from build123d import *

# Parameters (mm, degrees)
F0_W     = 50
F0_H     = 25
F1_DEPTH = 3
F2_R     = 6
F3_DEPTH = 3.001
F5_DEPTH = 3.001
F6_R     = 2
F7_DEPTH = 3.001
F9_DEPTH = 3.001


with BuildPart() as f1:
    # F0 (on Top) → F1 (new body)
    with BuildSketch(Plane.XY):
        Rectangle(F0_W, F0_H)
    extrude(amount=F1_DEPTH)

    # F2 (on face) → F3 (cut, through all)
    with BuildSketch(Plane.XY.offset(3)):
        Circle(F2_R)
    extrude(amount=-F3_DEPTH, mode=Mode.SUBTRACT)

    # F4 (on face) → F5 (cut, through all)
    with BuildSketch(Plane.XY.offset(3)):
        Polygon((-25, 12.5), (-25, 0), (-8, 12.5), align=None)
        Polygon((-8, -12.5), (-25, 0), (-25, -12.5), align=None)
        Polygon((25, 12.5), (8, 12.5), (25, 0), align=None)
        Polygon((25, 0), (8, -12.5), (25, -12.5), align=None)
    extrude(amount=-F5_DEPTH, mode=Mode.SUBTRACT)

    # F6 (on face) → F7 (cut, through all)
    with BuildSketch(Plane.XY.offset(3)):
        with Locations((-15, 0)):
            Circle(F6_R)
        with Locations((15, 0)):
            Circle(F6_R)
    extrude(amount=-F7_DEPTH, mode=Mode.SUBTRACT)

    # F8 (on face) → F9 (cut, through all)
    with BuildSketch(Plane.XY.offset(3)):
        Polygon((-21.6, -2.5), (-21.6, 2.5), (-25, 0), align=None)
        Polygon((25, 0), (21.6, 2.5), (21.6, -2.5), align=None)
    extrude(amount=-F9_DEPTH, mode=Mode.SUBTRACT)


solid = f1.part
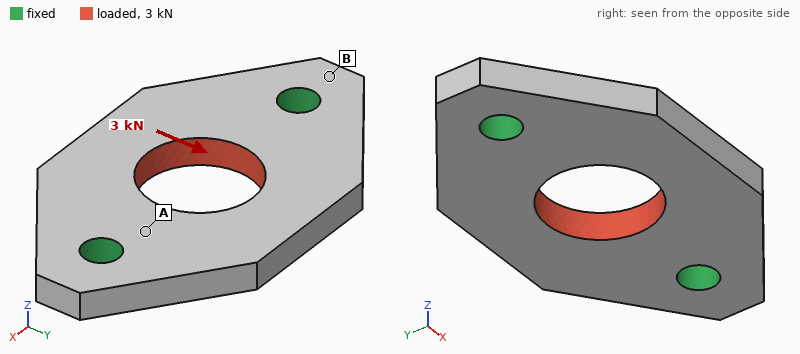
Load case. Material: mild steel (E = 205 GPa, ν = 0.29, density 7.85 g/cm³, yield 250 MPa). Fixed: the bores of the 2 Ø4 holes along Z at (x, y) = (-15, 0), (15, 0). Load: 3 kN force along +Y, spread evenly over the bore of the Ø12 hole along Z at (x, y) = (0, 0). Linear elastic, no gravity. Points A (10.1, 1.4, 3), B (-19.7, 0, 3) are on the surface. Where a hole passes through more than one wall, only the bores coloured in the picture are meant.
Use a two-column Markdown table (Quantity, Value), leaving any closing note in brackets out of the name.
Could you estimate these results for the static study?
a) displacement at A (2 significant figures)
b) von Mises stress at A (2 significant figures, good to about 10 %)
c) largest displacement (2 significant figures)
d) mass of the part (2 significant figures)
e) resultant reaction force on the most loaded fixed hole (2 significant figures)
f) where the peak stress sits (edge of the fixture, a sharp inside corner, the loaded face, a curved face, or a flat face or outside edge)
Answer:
| Quantity | Value |
|---|---|
| displacement at A | 2.2 µm |
| von Mises stress at A | 55 MPa |
| largest displacement | 5.6 µm |
| mass of the part | 16 g |
| resultant reaction force on the most loaded fixed hole | 1.5 kN |
| where the peak stress sits | edge of the fixture |
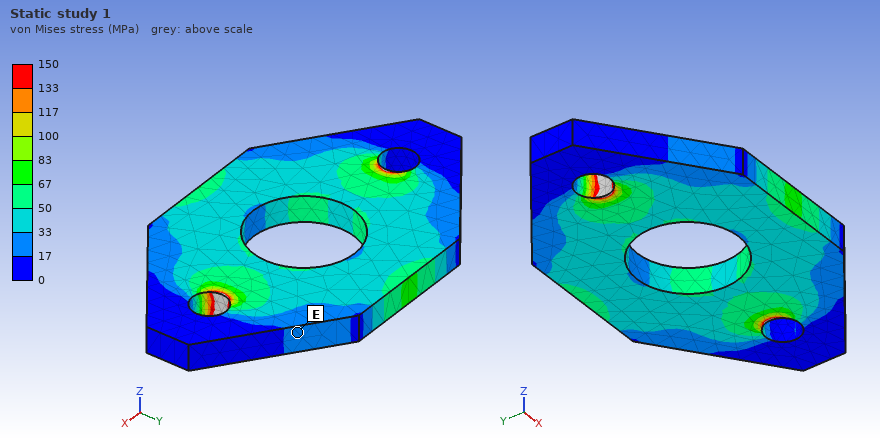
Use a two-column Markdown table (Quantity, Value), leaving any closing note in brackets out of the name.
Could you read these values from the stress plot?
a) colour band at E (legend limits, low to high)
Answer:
| Quantity | Value |
|---|---|
| colour band at E | 17 to 33 MPa |
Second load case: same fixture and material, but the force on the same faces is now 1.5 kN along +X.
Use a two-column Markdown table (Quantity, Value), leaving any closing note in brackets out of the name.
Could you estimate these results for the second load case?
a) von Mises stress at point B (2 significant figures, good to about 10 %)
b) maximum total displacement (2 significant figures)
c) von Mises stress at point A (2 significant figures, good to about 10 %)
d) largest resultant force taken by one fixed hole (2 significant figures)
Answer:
| Quantity | Value |
|---|---|
| von Mises stress at point B | 7.7 MPa |
| maximum total displacement | 1.5 µm |
| von Mises stress at point A | 24 MPa |
| largest resultant force taken by one fixed hole | 750 N |
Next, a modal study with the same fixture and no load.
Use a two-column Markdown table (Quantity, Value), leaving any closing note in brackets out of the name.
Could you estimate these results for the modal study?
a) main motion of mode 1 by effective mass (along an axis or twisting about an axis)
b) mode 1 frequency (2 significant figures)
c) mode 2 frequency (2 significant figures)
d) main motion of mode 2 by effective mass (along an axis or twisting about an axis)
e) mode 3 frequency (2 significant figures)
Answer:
| Quantity | Value |
|---|---|
| main motion of mode 1 by effective mass | twisting about X |
| mode 1 frequency | 12 kHz |
| mode 2 frequency | 13 kHz |
| main motion of mode 2 by effective mass | along Z |
| mode 3 frequency | 28 kHz |
